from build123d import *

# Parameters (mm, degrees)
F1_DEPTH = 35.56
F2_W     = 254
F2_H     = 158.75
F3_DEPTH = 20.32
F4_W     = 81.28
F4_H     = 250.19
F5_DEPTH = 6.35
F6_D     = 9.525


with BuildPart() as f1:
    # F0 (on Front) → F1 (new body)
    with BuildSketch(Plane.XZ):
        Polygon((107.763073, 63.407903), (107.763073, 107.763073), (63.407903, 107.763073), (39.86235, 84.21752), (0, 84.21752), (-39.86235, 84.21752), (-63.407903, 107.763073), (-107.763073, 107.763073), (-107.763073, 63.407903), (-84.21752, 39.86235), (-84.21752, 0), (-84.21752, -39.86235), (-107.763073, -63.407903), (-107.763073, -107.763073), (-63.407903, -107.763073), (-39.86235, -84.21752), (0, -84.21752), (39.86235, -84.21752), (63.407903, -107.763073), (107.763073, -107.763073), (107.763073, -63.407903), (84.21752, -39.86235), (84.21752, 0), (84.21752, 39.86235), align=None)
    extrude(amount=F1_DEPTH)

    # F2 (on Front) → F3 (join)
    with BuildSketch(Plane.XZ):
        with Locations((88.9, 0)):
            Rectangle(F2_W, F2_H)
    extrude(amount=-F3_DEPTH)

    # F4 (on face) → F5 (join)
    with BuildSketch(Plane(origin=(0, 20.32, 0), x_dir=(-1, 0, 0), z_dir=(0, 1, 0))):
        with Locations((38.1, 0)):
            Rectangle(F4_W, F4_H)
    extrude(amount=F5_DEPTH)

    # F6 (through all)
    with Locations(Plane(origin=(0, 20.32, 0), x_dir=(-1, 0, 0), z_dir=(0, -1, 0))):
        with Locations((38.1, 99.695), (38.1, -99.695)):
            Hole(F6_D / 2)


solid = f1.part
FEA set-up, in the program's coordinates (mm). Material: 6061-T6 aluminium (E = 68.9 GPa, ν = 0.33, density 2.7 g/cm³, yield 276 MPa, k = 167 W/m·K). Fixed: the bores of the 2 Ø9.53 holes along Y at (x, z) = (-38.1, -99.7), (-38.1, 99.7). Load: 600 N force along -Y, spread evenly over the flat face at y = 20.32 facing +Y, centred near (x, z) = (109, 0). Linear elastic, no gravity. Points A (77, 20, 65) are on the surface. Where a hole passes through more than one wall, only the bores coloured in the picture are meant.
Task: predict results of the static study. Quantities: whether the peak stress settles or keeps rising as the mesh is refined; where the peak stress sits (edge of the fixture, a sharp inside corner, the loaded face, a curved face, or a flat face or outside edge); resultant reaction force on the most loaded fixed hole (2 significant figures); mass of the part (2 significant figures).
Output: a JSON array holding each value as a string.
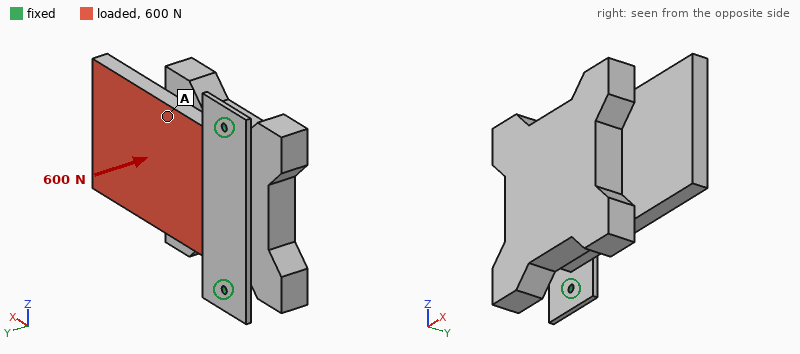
["keeps rising", "edge of the fixture", "410 N", "6.1 kg"]
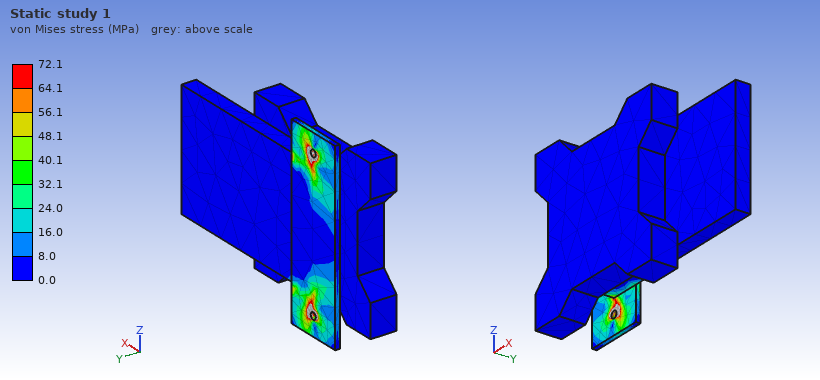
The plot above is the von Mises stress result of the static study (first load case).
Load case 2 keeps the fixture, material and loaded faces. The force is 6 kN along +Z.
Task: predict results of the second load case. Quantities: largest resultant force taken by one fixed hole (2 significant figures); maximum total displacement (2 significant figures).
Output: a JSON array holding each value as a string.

["5.4 kN", "84 µm"]
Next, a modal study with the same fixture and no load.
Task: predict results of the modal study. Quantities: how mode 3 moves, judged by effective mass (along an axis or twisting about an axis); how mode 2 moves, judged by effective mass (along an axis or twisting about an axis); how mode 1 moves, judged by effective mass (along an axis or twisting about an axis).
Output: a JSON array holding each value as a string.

["along Z", "along Y", "along Y"]
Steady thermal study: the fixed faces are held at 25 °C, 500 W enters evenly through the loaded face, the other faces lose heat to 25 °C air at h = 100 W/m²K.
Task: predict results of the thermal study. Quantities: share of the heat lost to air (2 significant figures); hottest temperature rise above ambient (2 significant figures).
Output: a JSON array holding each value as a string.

["86 %", "55 K"]
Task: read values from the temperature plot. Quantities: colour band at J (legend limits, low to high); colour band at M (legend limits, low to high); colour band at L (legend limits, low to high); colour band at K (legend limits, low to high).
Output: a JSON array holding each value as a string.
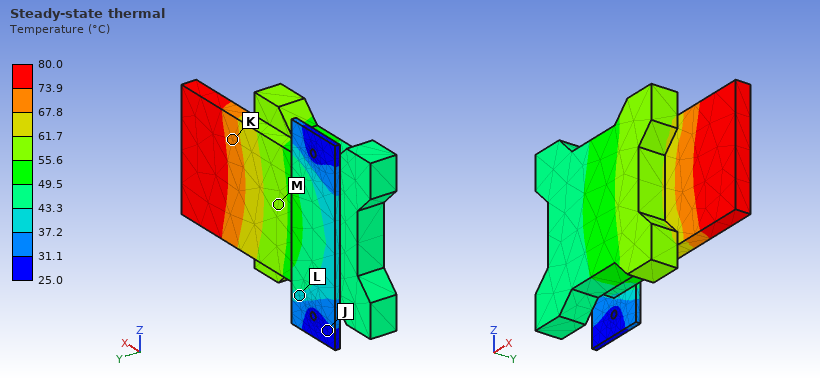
["25.0 to 31.1 °C", "55.6 to 61.7 °C", "37.2 to 43.3 °C", "67.8 to 73.9 °C"]
